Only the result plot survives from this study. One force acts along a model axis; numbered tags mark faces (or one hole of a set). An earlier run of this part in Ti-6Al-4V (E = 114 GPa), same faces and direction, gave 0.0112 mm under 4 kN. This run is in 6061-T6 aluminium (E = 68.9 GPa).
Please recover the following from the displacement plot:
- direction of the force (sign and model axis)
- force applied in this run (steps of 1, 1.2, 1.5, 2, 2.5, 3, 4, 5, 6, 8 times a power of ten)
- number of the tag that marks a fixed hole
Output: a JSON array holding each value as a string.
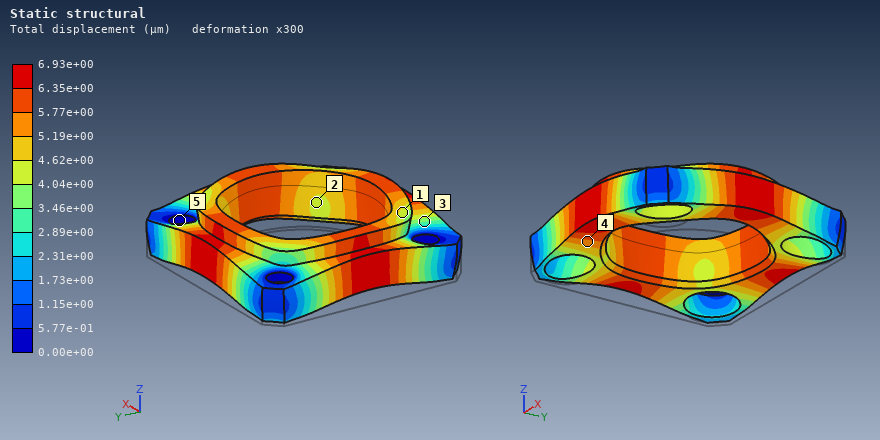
["+Z", "1.5 kN", "5"]
